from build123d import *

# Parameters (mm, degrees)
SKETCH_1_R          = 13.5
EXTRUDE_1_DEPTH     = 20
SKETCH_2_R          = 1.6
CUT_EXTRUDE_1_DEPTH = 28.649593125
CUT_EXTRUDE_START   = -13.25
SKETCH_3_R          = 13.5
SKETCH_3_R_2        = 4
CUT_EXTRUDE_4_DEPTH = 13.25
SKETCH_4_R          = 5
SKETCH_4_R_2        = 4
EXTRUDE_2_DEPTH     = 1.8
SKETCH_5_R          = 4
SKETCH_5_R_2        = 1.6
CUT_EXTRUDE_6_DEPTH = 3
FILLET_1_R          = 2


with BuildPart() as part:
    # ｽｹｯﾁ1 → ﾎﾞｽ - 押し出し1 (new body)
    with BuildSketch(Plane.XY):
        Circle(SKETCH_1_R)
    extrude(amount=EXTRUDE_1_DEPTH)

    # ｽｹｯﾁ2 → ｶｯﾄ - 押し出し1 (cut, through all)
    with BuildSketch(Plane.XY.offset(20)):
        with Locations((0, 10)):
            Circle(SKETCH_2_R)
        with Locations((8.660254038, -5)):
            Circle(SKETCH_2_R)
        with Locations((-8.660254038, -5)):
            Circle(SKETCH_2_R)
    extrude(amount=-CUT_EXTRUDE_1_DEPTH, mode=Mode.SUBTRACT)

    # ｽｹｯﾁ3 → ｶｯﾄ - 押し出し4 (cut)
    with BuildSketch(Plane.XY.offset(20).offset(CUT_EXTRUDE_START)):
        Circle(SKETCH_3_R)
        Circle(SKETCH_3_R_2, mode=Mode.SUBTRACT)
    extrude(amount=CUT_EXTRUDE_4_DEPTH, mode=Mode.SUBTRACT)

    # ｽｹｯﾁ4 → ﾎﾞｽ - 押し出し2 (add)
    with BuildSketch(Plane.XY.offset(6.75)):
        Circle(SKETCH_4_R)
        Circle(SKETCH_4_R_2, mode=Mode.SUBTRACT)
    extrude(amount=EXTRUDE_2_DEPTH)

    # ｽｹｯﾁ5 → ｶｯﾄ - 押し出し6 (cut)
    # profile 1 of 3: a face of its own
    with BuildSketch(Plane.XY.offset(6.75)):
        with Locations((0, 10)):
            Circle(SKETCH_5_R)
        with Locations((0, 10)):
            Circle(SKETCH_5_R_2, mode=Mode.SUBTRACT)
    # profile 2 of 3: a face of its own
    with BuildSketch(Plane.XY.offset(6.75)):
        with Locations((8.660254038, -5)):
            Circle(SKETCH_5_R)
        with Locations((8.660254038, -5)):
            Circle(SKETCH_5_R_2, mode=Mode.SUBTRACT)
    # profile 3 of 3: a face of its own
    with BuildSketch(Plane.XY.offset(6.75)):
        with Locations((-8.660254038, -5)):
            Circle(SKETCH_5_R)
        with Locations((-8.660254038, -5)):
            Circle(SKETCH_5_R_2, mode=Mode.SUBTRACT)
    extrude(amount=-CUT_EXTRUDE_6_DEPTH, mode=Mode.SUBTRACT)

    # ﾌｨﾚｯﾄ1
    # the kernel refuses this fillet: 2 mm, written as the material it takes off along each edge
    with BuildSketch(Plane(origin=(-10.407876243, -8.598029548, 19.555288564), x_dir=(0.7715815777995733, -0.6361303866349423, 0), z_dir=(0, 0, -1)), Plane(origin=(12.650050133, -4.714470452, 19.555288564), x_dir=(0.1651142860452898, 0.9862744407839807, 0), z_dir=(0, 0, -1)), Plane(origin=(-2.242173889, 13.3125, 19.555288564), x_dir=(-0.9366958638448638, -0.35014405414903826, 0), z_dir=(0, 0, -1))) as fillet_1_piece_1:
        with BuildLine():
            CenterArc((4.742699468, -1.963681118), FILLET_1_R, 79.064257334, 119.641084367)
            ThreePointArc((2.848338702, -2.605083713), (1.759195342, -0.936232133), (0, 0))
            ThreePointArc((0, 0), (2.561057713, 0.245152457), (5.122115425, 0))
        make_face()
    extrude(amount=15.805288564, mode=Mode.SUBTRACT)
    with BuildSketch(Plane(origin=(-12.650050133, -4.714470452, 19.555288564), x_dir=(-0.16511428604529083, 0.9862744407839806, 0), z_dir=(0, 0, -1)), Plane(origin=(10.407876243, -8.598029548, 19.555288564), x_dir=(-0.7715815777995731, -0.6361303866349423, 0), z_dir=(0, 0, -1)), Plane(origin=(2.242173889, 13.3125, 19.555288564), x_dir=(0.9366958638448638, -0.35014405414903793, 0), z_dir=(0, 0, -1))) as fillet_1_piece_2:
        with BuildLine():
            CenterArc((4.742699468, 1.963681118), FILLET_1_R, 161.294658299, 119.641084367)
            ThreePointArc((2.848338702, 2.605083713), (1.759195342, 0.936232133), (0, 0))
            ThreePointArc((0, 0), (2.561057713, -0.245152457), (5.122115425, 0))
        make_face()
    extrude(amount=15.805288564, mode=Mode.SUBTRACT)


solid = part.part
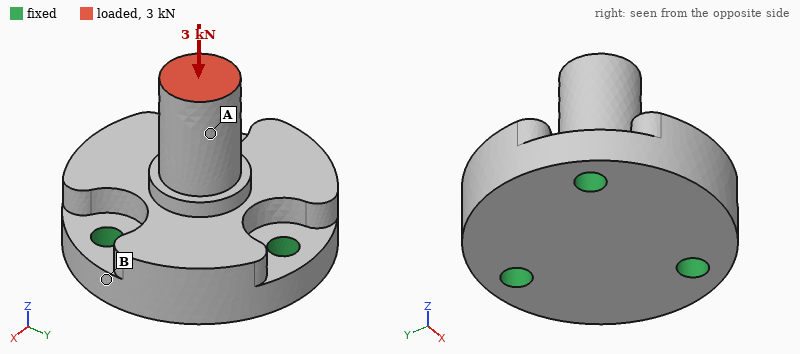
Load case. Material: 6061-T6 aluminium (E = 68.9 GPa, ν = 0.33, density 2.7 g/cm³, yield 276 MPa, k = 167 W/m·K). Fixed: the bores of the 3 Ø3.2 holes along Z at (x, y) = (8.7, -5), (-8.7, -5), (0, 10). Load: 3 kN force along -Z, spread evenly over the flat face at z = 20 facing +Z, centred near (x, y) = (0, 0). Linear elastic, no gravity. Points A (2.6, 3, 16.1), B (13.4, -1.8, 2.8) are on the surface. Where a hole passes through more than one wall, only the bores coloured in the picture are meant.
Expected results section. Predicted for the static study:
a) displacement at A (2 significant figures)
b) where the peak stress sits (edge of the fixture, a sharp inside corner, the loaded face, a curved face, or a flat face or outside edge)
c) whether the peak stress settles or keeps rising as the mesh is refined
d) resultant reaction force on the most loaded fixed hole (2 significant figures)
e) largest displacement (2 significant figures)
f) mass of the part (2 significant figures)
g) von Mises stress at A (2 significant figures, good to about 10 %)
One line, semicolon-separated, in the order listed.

16 µm; edge of the fixture; keeps rising; 1.1 kN; 19 µm; 11 g; 60 MPa
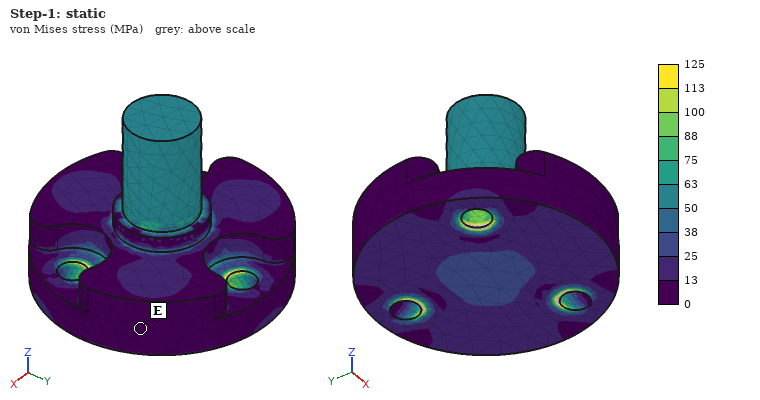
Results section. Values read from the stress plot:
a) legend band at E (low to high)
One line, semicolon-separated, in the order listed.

0 to 13 MPa
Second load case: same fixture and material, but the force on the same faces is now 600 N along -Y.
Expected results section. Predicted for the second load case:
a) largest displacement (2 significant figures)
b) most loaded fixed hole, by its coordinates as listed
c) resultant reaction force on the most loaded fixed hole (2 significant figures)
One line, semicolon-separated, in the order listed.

55 µm; (0, 10); 750 N
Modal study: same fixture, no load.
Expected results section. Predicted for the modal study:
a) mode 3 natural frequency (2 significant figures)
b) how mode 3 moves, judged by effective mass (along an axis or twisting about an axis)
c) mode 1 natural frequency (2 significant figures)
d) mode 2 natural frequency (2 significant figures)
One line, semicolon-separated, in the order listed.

38 kHz; along Z; 22 kHz; 22 kHz
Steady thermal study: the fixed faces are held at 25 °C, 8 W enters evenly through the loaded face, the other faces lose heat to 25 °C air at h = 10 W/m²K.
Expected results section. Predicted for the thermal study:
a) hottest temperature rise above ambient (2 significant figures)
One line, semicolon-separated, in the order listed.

15 K
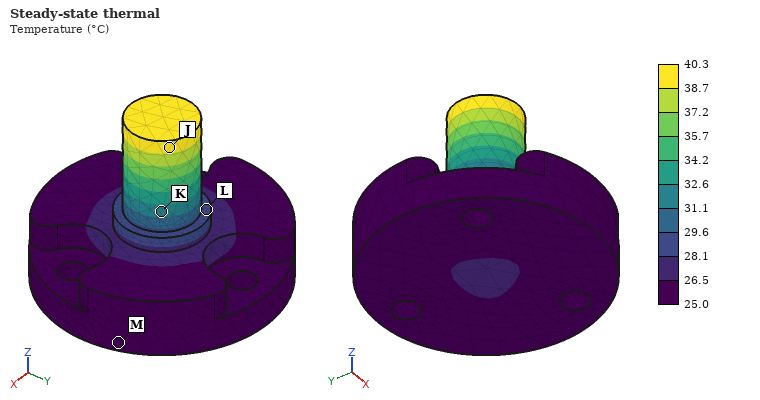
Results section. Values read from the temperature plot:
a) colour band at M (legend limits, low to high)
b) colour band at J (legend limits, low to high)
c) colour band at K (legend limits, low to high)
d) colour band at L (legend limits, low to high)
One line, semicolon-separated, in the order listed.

25.0 to 26.5 °C; 38.7 to 40.3 °C; 31.1 to 32.6 °C; 28.1 to 29.6 °C
